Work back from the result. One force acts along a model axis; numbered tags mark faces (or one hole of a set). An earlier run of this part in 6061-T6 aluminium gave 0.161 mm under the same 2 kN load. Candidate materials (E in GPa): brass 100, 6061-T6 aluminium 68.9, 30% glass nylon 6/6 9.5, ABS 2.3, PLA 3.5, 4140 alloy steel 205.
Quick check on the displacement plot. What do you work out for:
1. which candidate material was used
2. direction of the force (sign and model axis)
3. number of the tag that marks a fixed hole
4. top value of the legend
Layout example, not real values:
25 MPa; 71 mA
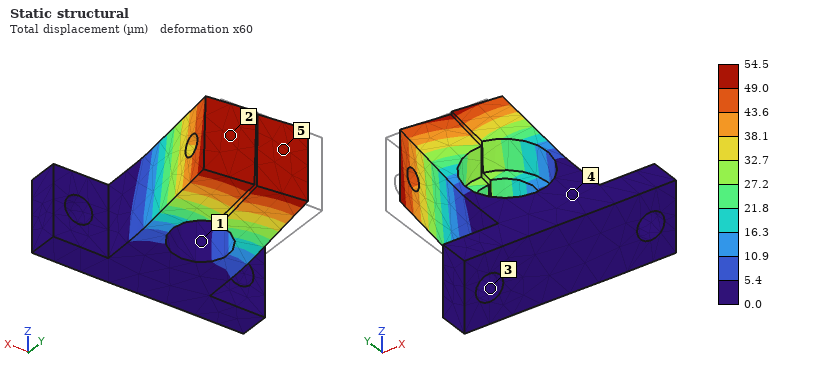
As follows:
4140 alloy steel; +X; 3; 54.5 µm
